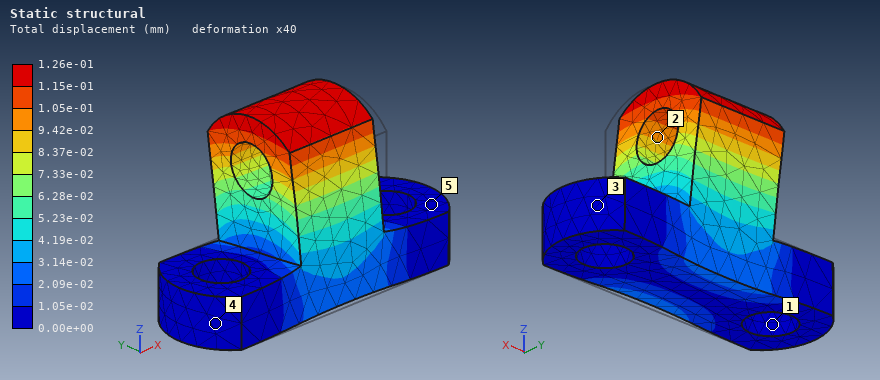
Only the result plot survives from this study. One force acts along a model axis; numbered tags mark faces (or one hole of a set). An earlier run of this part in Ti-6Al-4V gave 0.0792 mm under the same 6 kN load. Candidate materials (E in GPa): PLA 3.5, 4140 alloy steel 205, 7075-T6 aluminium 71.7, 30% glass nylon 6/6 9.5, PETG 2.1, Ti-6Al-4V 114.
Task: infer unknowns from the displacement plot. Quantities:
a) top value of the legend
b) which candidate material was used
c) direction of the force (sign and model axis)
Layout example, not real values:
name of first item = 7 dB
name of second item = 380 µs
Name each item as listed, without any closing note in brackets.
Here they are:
top value of the legend = 1.26e-01 mm
which candidate material was used = 7075-T6 aluminium
direction of the force = +Y
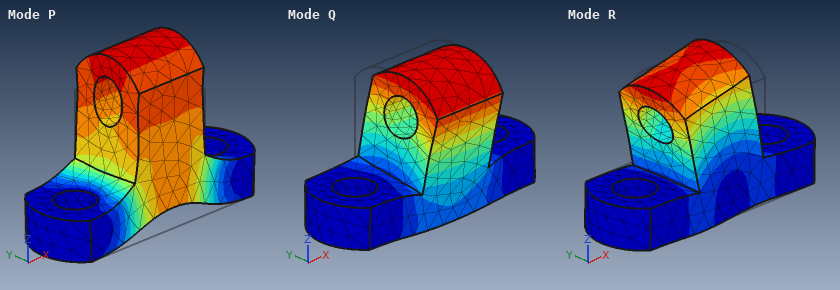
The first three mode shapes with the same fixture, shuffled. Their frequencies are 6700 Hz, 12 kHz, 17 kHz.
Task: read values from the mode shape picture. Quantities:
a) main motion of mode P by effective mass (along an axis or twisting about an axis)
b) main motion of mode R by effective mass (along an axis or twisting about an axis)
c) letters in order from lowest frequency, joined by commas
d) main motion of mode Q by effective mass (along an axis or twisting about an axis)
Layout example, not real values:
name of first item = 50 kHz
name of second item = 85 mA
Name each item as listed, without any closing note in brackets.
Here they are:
main motion of mode P by effective mass = along Z
main motion of mode R by effective mass = along X
letters in order from lowest frequency, joined by commas = Q, R, P
main motion of mode Q by effective mass = along Y
